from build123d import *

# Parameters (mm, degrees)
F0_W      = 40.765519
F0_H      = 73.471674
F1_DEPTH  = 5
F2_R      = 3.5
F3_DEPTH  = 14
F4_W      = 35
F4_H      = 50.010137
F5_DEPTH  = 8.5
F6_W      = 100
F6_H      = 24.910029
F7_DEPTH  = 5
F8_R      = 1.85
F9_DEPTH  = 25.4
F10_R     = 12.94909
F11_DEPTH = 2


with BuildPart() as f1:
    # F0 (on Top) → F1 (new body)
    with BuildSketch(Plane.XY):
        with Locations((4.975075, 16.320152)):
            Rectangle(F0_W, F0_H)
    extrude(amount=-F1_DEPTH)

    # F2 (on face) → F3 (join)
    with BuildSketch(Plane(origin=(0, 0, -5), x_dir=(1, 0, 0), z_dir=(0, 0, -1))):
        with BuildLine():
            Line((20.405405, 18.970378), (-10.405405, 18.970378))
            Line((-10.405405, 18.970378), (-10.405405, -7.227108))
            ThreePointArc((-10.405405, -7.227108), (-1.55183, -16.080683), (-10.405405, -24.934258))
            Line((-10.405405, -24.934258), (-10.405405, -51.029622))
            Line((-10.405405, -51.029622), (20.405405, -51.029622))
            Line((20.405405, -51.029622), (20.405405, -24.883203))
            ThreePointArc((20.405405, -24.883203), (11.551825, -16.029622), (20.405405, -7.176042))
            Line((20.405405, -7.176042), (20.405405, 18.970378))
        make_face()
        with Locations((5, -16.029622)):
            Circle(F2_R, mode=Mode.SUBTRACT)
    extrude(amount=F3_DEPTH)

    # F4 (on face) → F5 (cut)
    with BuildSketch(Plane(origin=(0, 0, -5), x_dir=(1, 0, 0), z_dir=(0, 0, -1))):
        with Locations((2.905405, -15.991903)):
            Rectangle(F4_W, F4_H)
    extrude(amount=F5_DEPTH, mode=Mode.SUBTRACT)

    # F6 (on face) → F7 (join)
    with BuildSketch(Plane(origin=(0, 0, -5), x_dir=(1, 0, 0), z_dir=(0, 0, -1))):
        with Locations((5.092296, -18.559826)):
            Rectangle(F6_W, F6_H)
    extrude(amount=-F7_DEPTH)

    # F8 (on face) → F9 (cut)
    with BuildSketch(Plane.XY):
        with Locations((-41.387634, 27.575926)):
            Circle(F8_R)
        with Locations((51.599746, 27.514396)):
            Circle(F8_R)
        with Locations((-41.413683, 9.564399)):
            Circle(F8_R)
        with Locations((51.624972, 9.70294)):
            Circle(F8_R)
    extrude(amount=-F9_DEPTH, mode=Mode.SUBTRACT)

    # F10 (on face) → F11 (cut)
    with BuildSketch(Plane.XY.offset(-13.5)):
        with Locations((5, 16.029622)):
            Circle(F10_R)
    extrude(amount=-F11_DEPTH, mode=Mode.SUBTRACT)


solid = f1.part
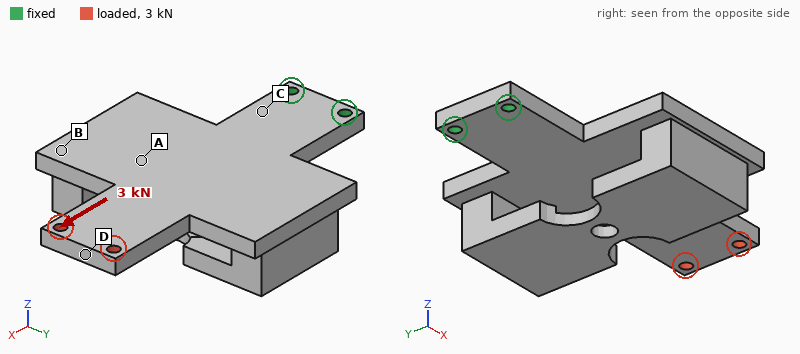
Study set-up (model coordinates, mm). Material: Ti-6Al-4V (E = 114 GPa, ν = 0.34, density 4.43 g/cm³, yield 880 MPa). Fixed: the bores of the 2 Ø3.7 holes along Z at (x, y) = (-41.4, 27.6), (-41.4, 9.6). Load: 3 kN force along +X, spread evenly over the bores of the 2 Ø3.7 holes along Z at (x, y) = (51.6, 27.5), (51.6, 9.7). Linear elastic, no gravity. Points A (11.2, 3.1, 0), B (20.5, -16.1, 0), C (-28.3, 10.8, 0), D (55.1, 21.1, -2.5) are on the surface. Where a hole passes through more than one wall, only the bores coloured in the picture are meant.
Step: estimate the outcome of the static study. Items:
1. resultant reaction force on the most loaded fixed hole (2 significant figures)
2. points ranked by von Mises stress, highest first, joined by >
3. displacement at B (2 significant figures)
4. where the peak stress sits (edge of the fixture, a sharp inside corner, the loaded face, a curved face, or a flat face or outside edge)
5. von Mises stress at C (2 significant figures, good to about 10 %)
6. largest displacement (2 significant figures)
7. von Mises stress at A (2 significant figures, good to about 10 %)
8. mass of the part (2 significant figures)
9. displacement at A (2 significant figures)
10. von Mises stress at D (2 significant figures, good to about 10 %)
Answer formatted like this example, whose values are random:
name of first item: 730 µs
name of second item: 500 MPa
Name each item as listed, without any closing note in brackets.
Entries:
resultant reaction force on the most loaded fixed hole: 1.5 kN
points ranked by von Mises stress, highest first, joined by >: D > C > A > B
displacement at B: 9.0 µm
where the peak stress sits: the loaded face
von Mises stress at C: 25 MPa
largest displacement: 22 µm
von Mises stress at A: 11 MPa
mass of the part: 160 g
displacement at A: 9.8 µm
von Mises stress at D: 32 MPa
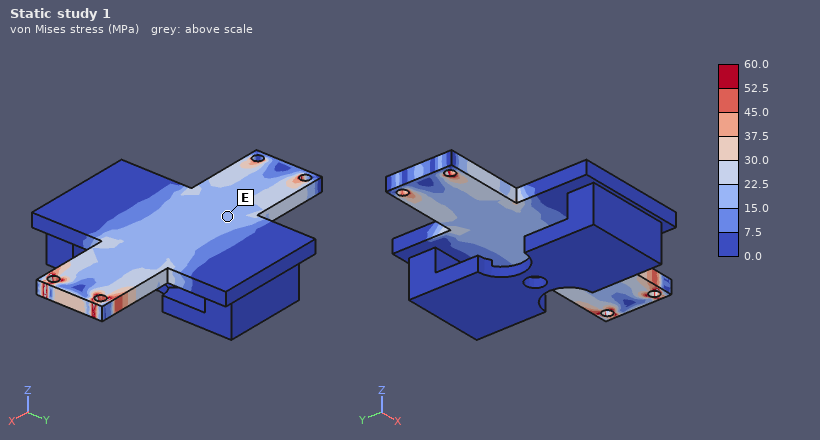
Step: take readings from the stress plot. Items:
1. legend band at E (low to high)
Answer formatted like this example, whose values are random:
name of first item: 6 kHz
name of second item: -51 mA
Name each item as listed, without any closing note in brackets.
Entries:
legend band at E: 15.0 to 22.5 MPa
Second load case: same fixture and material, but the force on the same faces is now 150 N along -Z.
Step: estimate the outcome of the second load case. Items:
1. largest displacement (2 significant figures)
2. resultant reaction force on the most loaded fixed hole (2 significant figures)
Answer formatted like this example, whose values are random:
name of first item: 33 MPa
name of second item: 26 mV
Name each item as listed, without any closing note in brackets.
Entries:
largest displacement: 1.2 mm
resultant reaction force on the most loaded fixed hole: 76 N
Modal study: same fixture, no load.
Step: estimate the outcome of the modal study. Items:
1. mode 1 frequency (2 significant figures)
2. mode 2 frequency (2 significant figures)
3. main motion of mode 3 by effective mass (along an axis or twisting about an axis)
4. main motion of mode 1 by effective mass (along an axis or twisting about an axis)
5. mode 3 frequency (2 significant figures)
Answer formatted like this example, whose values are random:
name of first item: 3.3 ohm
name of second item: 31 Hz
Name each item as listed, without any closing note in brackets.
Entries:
mode 1 frequency: 320 Hz
mode 2 frequency: 680 Hz
main motion of mode 3 by effective mass: along Y
main motion of mode 1 by effective mass: along Z
mode 3 frequency: 1400 Hz
